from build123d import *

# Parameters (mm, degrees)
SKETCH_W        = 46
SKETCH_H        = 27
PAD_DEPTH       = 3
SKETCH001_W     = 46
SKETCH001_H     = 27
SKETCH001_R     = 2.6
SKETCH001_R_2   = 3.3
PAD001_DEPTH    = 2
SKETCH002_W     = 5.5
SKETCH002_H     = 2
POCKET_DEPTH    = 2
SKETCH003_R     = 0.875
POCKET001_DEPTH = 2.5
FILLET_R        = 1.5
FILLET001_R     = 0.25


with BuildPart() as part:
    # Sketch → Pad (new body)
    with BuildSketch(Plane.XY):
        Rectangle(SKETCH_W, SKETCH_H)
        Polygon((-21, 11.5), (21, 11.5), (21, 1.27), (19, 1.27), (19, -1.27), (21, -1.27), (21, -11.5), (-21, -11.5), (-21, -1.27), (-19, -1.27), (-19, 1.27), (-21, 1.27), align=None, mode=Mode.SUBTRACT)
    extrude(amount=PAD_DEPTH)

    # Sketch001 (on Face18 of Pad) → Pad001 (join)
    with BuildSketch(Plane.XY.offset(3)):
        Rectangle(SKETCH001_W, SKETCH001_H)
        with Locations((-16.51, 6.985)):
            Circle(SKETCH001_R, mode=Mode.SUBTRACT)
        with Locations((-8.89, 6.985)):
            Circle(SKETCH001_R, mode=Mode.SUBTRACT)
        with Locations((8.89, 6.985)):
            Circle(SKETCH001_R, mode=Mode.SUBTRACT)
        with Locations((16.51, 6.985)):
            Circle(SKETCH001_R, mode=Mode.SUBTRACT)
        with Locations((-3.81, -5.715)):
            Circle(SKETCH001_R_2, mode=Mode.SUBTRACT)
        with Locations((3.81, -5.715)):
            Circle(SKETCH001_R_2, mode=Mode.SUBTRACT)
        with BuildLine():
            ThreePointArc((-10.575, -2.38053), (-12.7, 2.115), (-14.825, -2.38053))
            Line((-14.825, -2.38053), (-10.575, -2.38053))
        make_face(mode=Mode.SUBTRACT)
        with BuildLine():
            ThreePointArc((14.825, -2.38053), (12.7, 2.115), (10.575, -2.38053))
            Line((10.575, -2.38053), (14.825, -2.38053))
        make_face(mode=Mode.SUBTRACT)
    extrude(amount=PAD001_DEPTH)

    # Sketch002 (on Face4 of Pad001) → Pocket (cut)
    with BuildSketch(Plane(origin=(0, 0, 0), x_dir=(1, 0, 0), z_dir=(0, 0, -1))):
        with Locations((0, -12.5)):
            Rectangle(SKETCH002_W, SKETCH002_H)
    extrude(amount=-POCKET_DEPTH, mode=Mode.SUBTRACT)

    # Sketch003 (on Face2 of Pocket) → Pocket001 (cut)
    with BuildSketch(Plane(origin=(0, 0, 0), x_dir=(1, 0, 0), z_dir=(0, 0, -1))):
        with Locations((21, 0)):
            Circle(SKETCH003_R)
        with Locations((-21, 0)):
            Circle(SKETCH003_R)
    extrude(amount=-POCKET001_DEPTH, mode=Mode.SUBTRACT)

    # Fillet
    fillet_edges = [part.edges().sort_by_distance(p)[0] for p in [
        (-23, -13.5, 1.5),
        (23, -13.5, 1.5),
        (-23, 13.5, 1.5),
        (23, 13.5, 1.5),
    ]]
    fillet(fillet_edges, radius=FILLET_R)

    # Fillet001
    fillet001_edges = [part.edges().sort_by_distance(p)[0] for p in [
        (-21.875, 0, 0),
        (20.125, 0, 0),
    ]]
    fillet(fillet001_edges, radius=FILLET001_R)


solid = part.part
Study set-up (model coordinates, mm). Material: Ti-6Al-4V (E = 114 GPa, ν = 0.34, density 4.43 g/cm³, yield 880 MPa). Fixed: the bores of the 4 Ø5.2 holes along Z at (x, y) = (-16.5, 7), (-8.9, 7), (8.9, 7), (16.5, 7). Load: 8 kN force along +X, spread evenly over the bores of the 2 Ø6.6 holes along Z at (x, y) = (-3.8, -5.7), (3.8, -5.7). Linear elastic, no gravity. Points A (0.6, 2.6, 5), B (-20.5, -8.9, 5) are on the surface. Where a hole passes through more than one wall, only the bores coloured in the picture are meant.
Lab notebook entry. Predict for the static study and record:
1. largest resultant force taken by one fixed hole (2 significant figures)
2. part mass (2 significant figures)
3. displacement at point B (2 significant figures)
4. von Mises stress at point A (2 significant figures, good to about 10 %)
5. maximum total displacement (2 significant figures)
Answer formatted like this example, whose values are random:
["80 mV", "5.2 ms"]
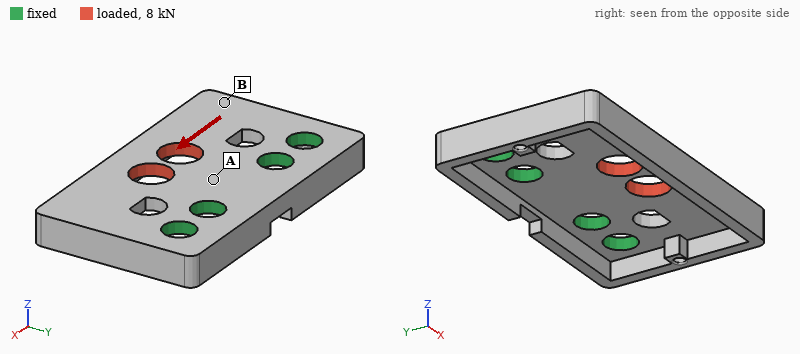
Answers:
["2.7 kN", "13 g", "52 µm", "190 MPa", "83 µm"]
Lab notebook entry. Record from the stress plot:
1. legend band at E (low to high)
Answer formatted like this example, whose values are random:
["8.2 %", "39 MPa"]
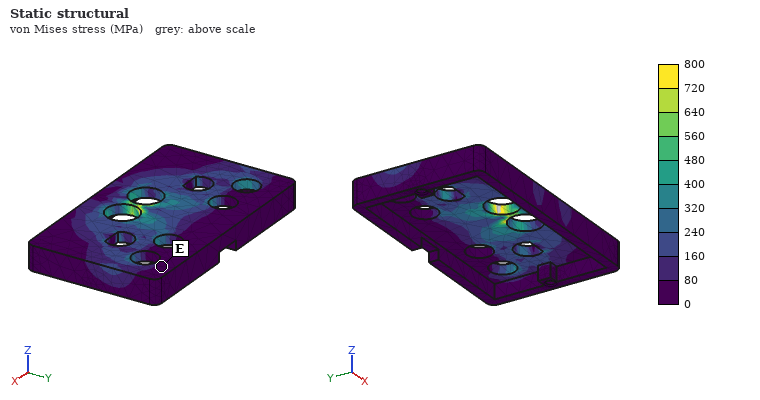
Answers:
["0 to 80 MPa"]
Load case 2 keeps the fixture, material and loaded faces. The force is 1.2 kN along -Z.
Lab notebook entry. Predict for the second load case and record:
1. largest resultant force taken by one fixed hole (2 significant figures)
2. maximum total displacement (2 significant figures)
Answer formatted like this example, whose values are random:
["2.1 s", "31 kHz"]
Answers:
["490 N", "0.26 mm"]
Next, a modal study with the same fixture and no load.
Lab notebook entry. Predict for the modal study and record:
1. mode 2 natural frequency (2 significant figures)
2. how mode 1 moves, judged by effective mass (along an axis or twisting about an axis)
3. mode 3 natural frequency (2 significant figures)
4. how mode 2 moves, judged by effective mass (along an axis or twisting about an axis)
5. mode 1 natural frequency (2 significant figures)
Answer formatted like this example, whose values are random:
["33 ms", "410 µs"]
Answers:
["6300 Hz", "along Z", "13 kHz", "twisting about Y", "4500 Hz"]
